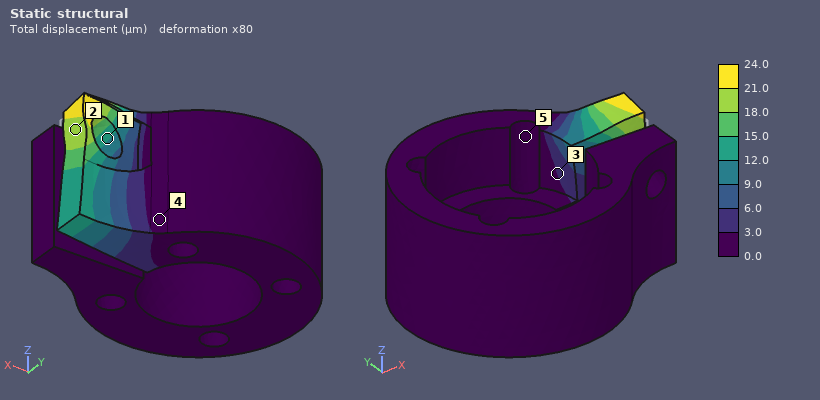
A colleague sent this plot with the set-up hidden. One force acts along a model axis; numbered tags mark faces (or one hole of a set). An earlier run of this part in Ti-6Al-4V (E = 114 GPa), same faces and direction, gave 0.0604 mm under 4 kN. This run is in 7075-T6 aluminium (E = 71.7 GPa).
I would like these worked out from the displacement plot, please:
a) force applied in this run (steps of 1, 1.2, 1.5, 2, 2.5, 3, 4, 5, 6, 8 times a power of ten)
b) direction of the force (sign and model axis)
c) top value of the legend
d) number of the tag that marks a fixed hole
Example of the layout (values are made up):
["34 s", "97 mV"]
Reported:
["1 kN", "+Z", "24.0 µm", "5"]
